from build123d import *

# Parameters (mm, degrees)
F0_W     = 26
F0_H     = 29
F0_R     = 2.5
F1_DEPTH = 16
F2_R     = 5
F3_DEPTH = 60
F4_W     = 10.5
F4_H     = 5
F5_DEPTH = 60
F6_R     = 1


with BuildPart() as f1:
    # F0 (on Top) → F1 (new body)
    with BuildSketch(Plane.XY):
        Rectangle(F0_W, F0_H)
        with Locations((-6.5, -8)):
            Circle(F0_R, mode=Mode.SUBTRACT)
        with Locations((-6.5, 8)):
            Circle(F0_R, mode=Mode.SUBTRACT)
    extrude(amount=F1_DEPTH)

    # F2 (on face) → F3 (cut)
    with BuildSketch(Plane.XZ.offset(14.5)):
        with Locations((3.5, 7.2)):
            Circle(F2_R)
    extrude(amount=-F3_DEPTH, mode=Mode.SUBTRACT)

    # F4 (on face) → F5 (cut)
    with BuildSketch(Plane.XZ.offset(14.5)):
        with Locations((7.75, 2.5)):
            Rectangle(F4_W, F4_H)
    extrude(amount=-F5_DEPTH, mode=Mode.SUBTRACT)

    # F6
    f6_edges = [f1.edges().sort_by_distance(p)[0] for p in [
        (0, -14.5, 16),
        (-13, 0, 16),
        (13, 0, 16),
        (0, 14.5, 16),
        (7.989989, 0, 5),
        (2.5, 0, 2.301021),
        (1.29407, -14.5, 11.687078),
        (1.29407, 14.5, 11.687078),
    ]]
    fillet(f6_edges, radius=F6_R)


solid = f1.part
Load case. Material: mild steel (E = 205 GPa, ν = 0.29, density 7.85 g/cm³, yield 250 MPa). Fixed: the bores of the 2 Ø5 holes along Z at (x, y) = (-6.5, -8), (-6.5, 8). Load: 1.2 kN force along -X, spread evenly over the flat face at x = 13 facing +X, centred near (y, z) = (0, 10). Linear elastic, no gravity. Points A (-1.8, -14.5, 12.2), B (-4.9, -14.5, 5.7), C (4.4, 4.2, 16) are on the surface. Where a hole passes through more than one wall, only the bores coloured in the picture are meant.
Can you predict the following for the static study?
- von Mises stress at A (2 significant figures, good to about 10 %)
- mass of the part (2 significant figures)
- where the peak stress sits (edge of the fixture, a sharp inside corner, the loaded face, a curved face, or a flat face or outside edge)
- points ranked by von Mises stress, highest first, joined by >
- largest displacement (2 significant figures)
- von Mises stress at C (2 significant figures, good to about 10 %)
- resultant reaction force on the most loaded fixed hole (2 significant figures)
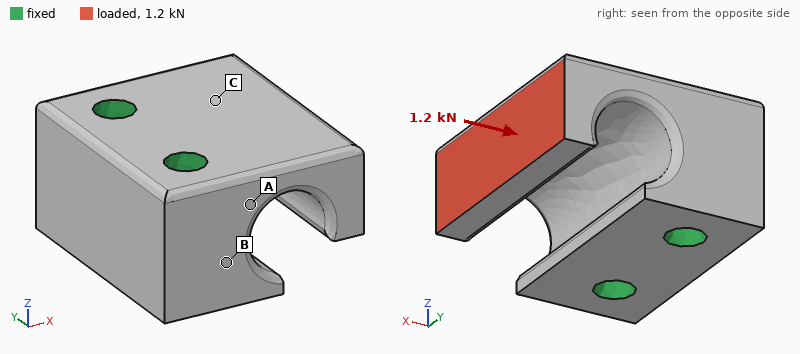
19 MPa
62 g
a curved face
C > A > B
17 µm
45 MPa
610 N
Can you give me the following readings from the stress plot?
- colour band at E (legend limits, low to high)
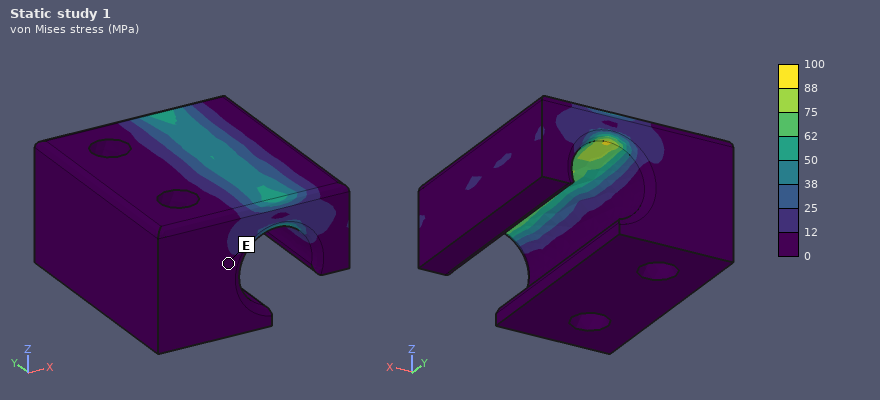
0 to 12 MPa
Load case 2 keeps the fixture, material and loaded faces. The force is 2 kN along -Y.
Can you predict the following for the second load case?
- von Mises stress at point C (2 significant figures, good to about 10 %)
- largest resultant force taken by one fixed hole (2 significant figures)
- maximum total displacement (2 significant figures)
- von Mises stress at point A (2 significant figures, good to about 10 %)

17 MPa
2.1 kN
13 µm
35 MPa
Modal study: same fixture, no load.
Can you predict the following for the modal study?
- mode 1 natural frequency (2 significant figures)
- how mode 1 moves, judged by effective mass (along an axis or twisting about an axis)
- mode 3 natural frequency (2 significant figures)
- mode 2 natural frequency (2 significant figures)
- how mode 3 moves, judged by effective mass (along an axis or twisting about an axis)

9100 Hz
along Z
26 kHz
16 kHz
along Y
